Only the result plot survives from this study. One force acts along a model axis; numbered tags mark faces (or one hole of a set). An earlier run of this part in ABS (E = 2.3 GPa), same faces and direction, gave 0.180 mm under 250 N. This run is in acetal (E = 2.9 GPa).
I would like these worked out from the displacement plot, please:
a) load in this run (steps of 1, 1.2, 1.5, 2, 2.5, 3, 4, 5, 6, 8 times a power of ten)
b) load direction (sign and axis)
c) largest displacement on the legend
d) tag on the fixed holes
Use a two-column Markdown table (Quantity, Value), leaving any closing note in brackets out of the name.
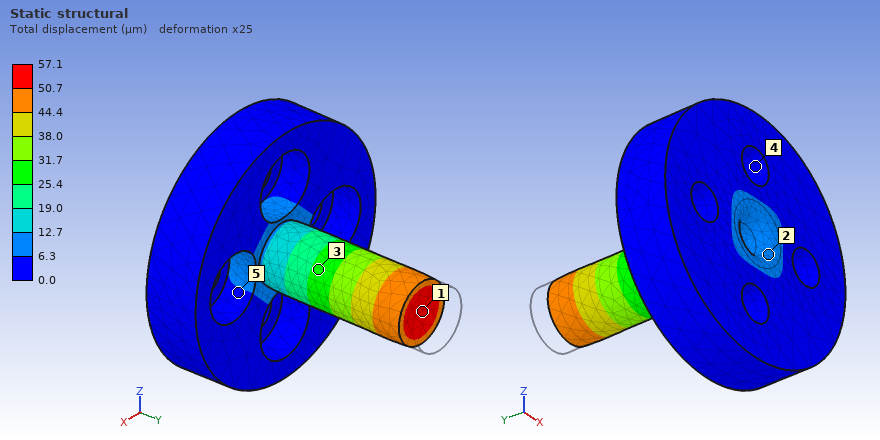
| Quantity | Value |
|---|---|
| load in this run | 100 N |
| load direction | -Y |
| largest displacement on the legend | 57.1 µm |
| tag on the fixed holes | 4 |
